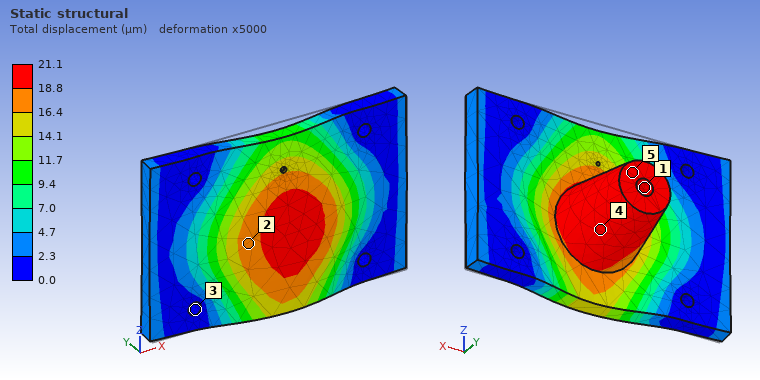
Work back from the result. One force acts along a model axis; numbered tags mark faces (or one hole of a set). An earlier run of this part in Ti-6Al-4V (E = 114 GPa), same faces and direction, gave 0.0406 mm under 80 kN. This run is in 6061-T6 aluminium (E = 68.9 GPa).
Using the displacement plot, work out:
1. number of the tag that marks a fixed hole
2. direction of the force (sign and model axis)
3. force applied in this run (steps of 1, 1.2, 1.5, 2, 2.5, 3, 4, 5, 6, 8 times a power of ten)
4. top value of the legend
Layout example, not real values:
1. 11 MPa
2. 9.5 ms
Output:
1. 3
2. -Y
3. 25 kN
4. 21.1 µm
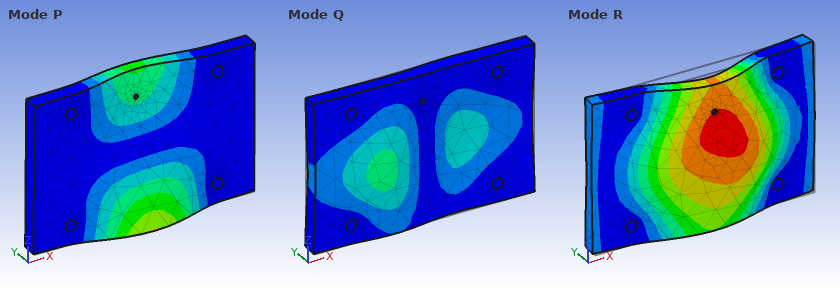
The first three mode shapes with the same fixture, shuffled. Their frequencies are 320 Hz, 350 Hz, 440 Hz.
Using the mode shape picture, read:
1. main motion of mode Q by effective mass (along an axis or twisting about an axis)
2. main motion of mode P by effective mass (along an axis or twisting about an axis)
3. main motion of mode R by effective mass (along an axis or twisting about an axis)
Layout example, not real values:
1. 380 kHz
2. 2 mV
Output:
1. along X
2. along Z
3. along Y
